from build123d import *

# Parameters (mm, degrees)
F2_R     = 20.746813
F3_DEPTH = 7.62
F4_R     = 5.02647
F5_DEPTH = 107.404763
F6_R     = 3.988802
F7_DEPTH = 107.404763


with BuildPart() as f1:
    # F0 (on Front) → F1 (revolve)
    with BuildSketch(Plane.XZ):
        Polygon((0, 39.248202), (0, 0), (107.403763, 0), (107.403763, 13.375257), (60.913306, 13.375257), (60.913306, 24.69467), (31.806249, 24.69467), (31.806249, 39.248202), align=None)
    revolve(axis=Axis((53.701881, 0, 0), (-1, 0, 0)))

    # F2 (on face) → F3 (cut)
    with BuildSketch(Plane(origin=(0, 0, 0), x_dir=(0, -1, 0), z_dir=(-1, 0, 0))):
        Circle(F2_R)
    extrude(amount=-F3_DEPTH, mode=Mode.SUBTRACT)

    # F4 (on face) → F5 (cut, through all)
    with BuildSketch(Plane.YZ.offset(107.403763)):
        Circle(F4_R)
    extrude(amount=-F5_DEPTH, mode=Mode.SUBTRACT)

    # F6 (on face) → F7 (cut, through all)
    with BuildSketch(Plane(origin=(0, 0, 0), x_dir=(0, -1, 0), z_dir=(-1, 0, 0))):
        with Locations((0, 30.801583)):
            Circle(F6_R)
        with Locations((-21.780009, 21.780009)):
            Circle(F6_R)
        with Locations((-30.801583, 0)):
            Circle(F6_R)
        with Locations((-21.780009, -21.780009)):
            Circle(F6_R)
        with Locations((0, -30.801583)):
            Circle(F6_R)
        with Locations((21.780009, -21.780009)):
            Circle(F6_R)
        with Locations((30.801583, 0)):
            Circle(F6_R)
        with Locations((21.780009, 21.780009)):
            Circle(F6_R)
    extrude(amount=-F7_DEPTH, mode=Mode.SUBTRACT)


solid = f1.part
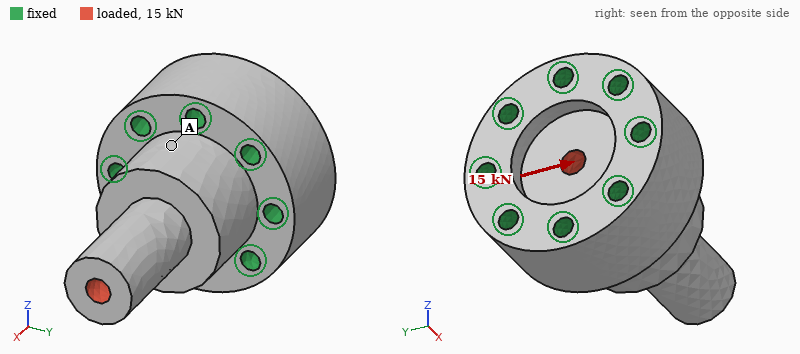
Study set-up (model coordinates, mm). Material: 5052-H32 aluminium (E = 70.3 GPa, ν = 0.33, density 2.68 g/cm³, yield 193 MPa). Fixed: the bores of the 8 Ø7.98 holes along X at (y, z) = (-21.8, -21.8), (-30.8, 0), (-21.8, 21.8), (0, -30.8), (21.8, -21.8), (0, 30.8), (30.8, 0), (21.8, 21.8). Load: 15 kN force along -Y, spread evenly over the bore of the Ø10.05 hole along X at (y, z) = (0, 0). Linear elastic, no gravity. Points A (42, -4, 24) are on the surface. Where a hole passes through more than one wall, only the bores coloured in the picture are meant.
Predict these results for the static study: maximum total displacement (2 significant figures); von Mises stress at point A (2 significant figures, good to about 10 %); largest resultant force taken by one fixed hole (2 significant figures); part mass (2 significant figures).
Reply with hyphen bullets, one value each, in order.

- 0.13 mm
- 8.2 MPa
- 5.9 kN
- 550 g
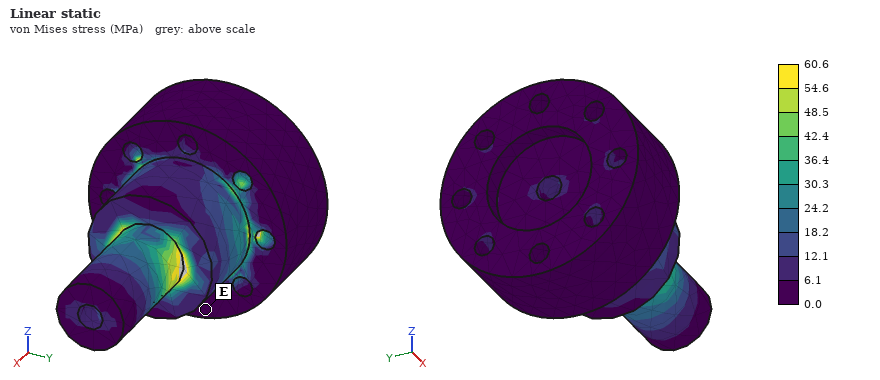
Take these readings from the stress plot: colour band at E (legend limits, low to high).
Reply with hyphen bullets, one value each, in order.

- 0.0 to 6.1 MPa
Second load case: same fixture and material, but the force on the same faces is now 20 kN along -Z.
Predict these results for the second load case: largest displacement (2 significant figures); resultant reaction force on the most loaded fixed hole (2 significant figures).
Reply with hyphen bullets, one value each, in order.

- 0.18 mm
- 7.9 kN
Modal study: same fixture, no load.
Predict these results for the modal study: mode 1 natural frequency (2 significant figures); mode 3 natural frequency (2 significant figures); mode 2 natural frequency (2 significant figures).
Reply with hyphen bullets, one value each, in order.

- 5700 Hz
- 15 kHz
- 5700 Hz
